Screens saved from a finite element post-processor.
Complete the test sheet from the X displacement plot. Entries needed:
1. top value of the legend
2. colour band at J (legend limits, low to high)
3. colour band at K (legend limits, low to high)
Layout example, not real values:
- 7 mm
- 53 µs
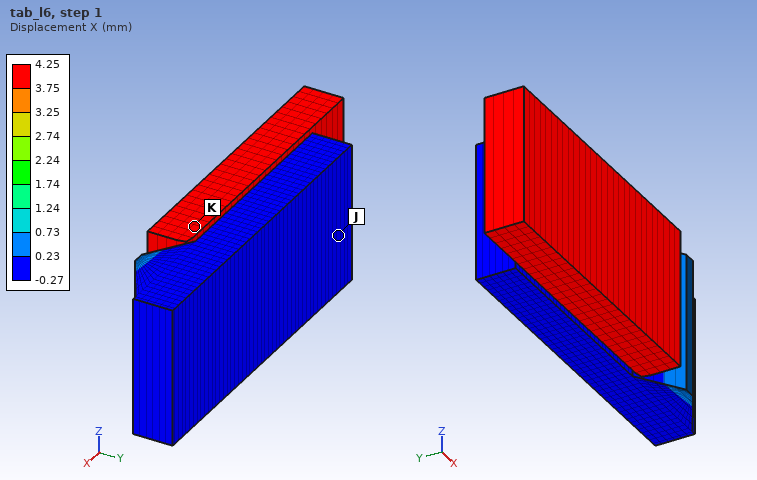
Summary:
- 4.25 mm
- -0.27 to 0.23 mm
- 3.75 to 4.25 mm
